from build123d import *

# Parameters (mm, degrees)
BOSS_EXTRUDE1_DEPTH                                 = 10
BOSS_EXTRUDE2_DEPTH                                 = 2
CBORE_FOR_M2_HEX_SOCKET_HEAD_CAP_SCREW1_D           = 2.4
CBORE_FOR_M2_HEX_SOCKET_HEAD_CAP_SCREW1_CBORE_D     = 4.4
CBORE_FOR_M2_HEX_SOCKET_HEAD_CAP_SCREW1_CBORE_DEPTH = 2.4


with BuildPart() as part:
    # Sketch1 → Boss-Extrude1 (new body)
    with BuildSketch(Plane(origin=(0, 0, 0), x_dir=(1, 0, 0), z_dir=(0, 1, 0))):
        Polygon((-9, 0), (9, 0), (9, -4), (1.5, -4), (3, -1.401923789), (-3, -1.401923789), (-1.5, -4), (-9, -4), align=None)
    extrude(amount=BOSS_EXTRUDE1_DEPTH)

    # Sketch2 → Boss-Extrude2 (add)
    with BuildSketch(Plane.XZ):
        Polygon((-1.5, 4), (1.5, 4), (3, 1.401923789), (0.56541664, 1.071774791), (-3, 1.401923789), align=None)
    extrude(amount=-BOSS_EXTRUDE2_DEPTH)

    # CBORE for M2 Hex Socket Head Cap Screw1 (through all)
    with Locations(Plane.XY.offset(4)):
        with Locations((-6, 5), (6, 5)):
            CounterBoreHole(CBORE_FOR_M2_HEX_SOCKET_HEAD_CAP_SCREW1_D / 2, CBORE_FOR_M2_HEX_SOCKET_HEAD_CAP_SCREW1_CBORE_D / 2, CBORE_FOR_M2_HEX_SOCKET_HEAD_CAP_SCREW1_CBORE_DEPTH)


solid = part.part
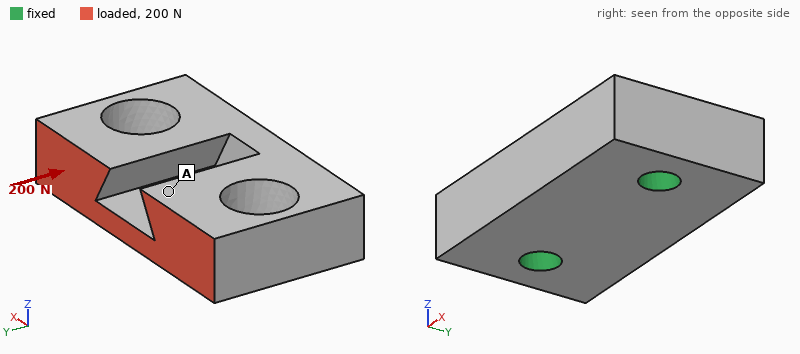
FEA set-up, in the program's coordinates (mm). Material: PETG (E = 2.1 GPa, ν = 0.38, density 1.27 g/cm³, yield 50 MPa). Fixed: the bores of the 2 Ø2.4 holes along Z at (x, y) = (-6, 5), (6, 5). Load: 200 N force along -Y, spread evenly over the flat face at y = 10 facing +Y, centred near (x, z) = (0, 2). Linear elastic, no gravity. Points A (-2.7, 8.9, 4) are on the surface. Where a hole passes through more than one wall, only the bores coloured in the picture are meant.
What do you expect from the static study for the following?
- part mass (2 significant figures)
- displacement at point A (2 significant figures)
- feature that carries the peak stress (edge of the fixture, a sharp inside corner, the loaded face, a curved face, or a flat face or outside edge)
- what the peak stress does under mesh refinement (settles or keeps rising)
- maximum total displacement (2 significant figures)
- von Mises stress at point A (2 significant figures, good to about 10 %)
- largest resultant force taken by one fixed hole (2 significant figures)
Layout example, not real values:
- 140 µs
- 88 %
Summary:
- 0.68 g
- 66 µm
- edge of the fixture
- keeps rising
- 80 µm
- 4.2 MPa
- 100 N
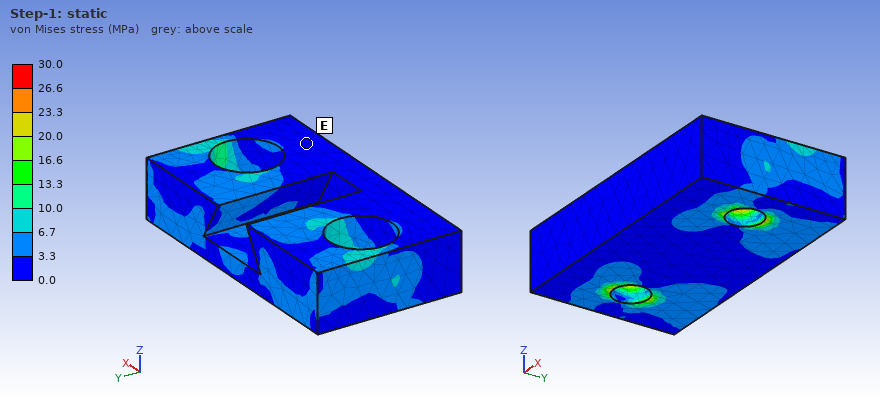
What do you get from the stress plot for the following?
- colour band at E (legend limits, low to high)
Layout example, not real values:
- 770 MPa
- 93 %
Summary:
- 0.0 to 3.3 MPa
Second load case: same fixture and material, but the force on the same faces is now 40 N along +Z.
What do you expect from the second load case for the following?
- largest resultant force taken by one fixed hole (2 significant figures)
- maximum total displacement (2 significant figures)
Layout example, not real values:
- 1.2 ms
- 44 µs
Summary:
- 20 N
- 71 µm
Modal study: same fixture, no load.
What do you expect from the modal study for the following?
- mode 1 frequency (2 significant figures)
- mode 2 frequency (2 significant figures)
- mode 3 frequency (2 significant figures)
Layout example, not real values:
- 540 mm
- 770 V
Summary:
- 8700 Hz
- 12 kHz
- 12 kHz
